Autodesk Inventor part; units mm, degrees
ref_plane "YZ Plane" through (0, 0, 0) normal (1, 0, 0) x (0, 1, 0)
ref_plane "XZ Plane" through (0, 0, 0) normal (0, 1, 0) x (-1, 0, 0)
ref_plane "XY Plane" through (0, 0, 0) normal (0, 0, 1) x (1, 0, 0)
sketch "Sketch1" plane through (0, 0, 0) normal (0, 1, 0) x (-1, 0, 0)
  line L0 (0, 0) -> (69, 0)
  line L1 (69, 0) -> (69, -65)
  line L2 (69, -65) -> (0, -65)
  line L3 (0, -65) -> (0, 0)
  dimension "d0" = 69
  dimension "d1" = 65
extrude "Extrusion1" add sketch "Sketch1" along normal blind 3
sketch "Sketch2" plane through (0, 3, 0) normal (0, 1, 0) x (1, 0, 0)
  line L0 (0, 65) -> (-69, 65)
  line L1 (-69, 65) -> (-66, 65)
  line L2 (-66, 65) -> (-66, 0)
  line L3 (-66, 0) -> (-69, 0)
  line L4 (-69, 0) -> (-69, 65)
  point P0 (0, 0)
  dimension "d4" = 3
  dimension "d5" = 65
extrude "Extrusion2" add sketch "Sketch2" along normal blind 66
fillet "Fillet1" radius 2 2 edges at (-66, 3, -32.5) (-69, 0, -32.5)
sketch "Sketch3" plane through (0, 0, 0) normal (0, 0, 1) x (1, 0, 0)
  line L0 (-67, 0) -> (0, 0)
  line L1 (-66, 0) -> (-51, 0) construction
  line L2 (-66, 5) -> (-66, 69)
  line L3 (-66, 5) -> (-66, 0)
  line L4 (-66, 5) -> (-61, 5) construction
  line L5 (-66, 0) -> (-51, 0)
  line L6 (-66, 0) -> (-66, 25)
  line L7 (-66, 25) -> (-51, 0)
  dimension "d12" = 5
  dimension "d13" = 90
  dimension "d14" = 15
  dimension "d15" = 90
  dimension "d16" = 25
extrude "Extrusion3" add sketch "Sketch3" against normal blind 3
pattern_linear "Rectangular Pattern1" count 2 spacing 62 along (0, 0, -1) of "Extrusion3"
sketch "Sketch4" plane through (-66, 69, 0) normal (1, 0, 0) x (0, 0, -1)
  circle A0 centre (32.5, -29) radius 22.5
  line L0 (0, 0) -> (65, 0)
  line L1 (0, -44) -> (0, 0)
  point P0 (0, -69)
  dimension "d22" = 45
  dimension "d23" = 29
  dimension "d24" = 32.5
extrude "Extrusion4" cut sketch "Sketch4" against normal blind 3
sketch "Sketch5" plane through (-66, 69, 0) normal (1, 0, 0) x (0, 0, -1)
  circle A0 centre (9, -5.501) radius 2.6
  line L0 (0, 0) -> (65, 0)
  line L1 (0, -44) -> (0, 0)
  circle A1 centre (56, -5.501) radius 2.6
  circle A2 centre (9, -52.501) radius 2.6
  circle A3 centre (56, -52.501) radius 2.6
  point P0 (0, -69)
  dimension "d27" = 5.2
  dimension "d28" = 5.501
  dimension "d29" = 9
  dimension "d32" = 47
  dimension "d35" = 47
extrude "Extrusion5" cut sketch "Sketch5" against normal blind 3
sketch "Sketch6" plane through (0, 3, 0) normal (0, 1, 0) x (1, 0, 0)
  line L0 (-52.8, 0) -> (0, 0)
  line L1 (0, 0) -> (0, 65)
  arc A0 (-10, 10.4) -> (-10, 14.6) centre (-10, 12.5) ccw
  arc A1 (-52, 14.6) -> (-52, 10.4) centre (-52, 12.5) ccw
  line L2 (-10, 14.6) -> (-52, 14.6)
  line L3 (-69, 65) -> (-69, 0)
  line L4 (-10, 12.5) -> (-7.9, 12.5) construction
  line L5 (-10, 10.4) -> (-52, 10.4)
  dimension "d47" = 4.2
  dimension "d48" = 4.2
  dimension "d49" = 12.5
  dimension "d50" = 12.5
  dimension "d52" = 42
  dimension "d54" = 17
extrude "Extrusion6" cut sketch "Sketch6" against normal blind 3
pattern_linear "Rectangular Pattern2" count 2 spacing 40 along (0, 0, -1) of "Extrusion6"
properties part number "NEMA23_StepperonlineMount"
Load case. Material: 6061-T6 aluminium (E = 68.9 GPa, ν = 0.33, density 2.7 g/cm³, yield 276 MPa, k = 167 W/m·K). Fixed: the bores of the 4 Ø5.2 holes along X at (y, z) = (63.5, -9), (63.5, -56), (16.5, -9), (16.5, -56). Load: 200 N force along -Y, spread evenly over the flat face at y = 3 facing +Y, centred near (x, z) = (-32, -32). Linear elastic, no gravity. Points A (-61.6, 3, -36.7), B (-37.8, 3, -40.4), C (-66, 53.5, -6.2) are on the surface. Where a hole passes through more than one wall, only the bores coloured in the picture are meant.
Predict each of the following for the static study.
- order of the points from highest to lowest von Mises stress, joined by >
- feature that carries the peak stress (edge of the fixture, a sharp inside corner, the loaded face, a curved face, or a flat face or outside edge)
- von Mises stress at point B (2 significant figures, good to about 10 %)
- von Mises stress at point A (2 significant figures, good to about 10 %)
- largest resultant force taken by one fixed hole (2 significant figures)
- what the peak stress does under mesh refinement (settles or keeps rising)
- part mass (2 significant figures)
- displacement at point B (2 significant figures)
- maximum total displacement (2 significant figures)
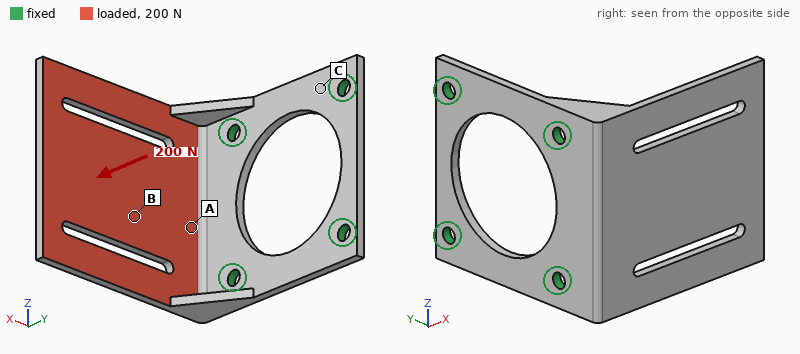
A > B > C
edge of the fixture
22 MPa
36 MPa
120 N
keeps rising
57 g
0.28 mm
0.89 mm
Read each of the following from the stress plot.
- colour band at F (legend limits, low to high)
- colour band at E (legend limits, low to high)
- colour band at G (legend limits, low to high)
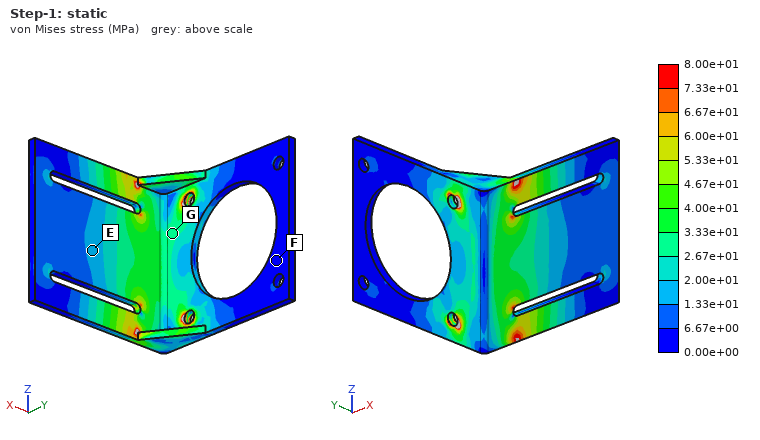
0.00e+00 to 6.67e+00 MPa
1.33e+01 to 2.00e+01 MPa
2.67e+01 to 3.33e+01 MPa
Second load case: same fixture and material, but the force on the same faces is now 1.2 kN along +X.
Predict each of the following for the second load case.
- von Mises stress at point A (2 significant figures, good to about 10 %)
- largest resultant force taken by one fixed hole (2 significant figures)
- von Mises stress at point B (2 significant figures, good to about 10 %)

14 MPa
630 N
14 MPa
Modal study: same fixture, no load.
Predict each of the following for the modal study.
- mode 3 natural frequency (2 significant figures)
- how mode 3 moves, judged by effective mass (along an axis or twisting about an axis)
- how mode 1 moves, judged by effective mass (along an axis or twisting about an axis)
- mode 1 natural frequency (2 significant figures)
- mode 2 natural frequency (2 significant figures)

2200 Hz
along Z
along Y
540 Hz
1400 Hz
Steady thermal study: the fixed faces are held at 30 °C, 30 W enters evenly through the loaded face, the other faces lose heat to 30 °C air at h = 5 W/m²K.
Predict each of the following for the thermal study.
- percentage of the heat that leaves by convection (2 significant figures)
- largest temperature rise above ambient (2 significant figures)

3.6 %
47 K
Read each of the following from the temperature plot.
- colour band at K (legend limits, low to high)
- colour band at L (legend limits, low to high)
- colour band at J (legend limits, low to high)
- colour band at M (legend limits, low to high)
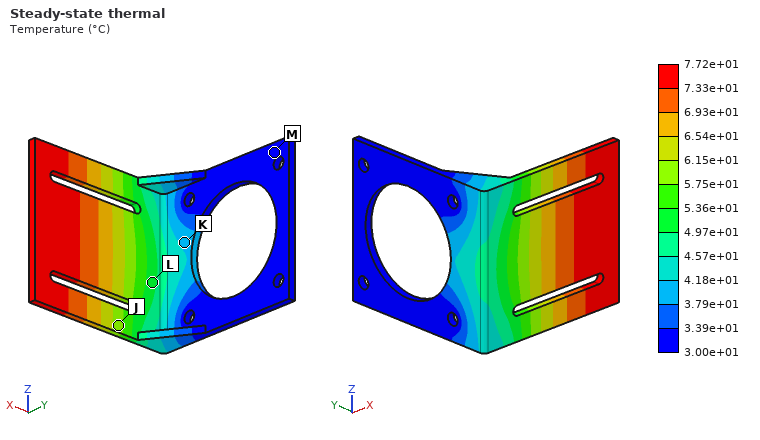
3.79e+01 to 4.18e+01 °C
4.97e+01 to 5.36e+01 °C
5.75e+01 to 6.15e+01 °C
3.00e+01 to 3.39e+01 °C
